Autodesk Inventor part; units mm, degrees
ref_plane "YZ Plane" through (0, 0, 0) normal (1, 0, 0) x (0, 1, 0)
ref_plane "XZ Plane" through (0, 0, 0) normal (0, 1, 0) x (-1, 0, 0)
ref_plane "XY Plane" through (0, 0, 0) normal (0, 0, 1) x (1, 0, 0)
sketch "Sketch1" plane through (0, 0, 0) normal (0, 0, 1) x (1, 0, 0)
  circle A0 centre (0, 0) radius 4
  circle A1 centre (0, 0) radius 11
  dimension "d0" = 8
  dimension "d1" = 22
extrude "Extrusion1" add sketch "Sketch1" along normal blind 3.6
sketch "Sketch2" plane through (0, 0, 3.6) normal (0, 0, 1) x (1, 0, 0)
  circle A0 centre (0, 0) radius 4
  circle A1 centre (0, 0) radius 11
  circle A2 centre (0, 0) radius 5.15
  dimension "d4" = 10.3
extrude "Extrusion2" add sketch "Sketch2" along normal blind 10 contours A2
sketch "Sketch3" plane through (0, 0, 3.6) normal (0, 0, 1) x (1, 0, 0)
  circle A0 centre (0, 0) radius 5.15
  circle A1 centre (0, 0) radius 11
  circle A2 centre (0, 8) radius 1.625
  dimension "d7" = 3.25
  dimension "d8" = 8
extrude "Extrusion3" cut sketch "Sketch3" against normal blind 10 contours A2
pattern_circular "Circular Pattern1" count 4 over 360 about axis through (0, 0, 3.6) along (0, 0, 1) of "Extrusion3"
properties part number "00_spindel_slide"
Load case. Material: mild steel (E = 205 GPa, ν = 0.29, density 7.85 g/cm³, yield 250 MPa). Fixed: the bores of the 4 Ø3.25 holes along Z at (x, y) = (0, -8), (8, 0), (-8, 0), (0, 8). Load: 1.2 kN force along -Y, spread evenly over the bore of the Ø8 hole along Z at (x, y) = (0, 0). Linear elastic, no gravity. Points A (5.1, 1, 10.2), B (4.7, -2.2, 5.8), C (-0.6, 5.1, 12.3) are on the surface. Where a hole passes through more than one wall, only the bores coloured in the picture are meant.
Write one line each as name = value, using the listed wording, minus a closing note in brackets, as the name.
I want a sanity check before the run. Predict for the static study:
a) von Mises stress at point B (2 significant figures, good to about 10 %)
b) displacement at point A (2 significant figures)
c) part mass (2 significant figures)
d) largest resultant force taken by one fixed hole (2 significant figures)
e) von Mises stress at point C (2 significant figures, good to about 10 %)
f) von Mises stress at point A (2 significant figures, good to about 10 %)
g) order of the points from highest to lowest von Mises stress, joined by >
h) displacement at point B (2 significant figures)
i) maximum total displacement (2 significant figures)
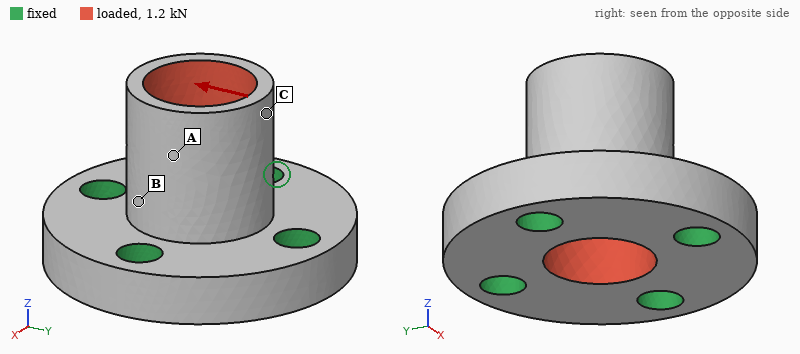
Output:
von Mises stress at point B = 49 MPa
displacement at point A = 5.1 µm
part mass = 11 g
largest resultant force taken by one fixed hole = 550 N
von Mises stress at point C = 14 MPa
von Mises stress at point A = 29 MPa
order of the points from highest to lowest von Mises stress, joined by > = B > A > C
displacement at point B = 2.3 µm
maximum total displacement = 7.4 µm
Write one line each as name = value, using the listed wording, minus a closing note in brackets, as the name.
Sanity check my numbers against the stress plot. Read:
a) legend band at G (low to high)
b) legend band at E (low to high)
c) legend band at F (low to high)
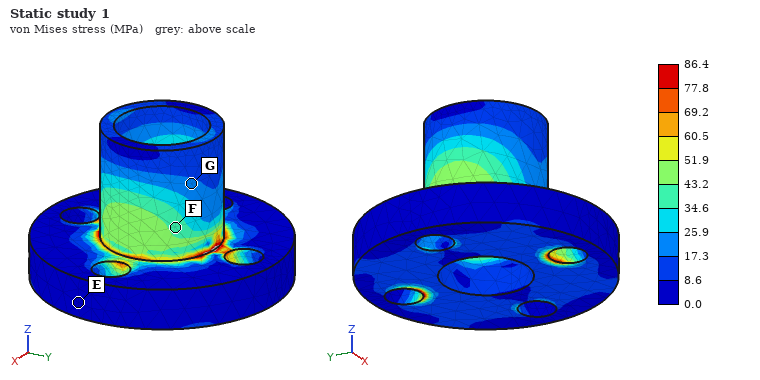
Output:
legend band at G = 17.3 to 25.9 MPa
legend band at E = 0.0 to 8.6 MPa
legend band at F = 34.6 to 43.2 MPa
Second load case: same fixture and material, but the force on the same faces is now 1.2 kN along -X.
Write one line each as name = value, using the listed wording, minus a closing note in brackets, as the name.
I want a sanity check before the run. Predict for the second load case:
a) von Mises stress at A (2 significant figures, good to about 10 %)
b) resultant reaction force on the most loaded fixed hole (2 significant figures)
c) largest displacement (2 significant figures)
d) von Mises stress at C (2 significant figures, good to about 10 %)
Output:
von Mises stress at A = 16 MPa
resultant reaction force on the most loaded fixed hole = 540 N
largest displacement = 7.5 µm
von Mises stress at C = 11 MPa
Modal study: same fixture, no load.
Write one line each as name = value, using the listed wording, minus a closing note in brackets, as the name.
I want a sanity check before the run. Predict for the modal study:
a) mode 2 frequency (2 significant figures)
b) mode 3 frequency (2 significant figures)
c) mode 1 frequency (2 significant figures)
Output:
mode 2 frequency = 40 kHz
mode 3 frequency = 43 kHz
mode 1 frequency = 40 kHz
